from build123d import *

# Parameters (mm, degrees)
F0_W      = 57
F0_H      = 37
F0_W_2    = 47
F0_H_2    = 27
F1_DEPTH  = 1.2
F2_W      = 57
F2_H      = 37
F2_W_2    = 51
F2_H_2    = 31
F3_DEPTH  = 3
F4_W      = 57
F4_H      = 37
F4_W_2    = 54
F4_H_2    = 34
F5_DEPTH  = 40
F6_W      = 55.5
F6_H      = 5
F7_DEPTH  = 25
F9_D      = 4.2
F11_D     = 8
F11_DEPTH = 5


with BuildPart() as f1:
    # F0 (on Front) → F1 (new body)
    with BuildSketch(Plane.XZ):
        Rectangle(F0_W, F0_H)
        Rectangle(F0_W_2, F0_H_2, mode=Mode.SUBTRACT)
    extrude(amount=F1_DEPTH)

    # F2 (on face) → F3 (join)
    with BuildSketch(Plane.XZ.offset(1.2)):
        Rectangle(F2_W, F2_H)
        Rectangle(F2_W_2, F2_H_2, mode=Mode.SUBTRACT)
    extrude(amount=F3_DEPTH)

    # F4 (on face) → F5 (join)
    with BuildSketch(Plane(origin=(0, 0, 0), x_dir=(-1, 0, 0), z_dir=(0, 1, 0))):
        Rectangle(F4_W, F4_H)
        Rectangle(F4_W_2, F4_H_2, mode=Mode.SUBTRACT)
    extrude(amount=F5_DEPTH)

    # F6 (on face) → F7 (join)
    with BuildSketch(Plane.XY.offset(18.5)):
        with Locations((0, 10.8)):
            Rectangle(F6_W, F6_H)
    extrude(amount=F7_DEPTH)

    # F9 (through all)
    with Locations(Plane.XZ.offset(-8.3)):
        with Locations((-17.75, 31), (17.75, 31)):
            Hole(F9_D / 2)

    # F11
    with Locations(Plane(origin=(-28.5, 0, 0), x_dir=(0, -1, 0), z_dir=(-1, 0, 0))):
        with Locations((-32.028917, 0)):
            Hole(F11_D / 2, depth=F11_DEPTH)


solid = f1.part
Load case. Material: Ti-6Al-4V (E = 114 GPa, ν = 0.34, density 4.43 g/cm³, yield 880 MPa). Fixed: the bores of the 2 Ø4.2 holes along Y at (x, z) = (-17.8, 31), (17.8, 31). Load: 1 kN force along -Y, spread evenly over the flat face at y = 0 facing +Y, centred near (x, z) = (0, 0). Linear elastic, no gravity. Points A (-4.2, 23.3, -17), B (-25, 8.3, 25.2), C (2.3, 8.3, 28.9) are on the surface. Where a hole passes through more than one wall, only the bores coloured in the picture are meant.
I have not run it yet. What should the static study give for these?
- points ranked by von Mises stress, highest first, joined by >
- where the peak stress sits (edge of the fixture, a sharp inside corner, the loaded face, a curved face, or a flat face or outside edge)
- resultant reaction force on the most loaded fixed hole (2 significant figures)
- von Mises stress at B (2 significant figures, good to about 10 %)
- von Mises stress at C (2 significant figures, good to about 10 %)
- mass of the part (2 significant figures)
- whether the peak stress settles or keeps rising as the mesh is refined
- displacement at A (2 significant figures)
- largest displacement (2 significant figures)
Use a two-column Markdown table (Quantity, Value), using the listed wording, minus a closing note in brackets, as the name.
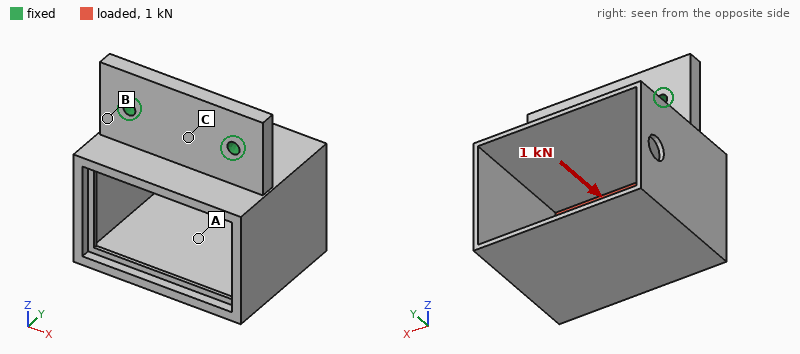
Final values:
| Quantity | Value |
|---|---|
| points ranked by von Mises stress, highest first, joined by > | B > C > A |
| where the peak stress sits | edge of the fixture |
| resultant reaction force on the most loaded fixed hole | 500 N |
| von Mises stress at B | 140 MPa |
| von Mises stress at C | 45 MPa |
| mass of the part | 90 g |
| whether the peak stress settles or keeps rising as the mesh is refined | keeps rising |
| displacement at A | 0.54 mm |
| largest displacement | 0.67 mm |
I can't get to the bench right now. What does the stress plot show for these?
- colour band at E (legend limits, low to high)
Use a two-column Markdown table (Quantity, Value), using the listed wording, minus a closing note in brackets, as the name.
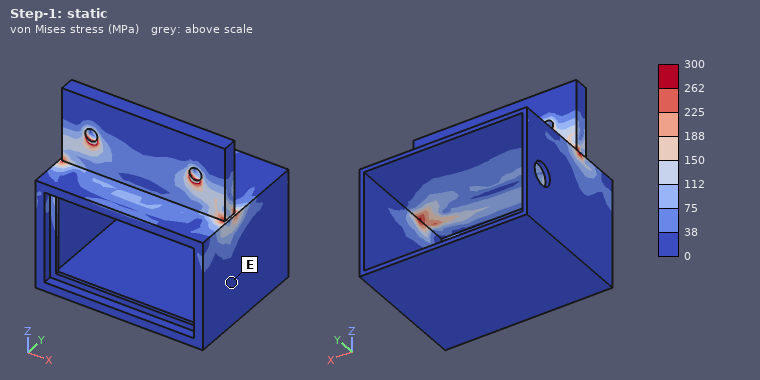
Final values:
| Quantity | Value |
|---|---|
| colour band at E | 0 to 38 MPa |
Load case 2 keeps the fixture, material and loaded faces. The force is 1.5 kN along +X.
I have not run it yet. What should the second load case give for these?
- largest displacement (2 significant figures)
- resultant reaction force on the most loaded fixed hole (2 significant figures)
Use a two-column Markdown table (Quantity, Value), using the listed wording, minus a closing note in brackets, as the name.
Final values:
| Quantity | Value |
|---|---|
| largest displacement | 0.53 mm |
| resultant reaction force on the most loaded fixed hole | 1.5 kN |
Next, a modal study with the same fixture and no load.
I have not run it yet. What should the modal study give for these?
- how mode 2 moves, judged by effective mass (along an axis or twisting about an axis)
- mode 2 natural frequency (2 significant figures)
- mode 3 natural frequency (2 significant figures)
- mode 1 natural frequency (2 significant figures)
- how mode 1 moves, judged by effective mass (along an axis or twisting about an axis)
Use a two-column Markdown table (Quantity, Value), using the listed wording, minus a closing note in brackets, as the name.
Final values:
| Quantity | Value |
|---|---|
| how mode 2 moves, judged by effective mass | along X |
| mode 2 natural frequency | 960 Hz |
| mode 3 natural frequency | 1700 Hz |
| mode 1 natural frequency | 870 Hz |
| how mode 1 moves, judged by effective mass | along Y |
